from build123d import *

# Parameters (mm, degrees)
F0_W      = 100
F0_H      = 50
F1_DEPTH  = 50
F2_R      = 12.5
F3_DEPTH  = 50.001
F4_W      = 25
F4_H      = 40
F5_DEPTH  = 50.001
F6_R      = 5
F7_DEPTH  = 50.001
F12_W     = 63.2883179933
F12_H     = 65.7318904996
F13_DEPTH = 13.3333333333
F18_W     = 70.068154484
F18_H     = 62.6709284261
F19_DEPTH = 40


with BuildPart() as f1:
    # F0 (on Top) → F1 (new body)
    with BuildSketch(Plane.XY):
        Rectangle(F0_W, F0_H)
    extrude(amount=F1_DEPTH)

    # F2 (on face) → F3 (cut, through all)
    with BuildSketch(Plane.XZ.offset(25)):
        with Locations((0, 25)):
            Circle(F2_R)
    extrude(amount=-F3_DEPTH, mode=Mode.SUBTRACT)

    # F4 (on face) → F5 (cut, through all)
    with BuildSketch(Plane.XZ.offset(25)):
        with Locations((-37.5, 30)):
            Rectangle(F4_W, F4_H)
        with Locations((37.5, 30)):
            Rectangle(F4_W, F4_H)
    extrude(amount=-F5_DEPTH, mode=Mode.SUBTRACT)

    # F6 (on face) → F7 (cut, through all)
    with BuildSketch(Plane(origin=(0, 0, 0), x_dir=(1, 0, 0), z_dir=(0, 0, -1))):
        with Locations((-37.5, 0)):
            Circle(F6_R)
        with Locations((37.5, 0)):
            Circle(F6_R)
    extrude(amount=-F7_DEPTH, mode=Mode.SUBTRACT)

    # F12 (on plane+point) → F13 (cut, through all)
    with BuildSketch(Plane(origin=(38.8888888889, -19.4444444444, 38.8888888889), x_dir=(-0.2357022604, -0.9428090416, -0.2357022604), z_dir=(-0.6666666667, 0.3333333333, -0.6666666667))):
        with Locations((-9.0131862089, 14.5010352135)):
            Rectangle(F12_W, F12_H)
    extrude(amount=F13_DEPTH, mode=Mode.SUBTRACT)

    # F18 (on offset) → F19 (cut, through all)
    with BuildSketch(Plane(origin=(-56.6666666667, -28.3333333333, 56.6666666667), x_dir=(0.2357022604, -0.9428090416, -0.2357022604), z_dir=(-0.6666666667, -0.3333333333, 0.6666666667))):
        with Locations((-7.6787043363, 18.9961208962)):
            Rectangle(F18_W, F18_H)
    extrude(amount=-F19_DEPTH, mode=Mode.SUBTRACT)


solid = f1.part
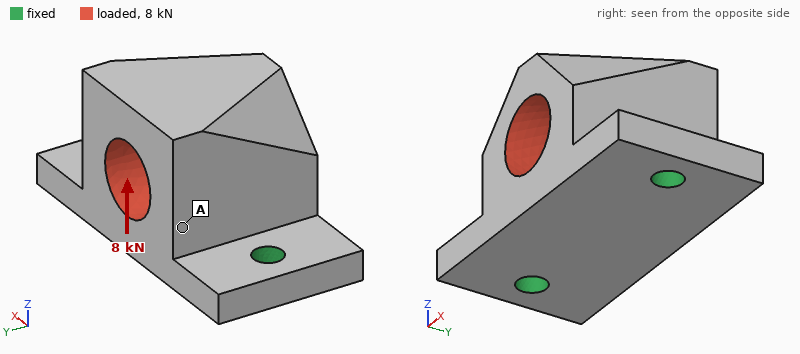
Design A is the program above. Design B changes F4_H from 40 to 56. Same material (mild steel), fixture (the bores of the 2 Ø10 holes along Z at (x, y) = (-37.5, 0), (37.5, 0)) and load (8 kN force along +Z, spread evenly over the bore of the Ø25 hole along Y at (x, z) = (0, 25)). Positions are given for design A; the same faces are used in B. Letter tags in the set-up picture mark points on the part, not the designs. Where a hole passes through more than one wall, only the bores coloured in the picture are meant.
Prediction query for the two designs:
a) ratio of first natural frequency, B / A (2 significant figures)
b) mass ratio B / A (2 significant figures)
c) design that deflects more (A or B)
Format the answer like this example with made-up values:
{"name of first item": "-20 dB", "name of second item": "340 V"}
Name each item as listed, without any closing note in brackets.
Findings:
{"ratio of first natural frequency, B / A": "0.14", "mass ratio B / A": "0.84", "design that deflects more": "B"}
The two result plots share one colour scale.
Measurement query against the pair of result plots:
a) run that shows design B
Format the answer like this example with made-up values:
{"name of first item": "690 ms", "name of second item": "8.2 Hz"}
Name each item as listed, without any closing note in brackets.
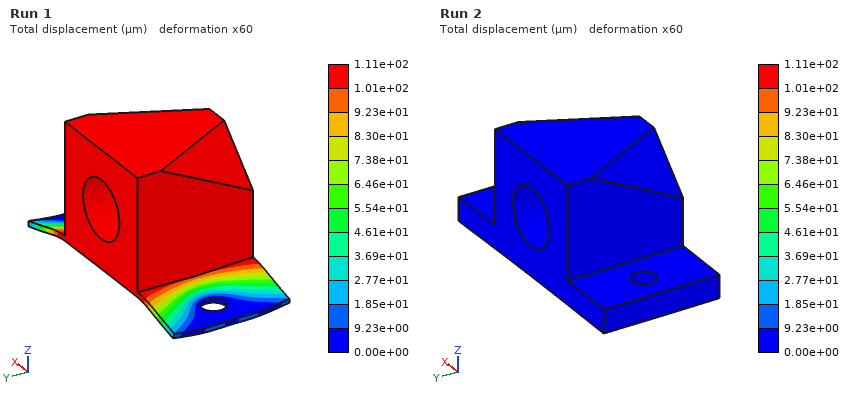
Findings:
{"run that shows design B": "Run 1"}
